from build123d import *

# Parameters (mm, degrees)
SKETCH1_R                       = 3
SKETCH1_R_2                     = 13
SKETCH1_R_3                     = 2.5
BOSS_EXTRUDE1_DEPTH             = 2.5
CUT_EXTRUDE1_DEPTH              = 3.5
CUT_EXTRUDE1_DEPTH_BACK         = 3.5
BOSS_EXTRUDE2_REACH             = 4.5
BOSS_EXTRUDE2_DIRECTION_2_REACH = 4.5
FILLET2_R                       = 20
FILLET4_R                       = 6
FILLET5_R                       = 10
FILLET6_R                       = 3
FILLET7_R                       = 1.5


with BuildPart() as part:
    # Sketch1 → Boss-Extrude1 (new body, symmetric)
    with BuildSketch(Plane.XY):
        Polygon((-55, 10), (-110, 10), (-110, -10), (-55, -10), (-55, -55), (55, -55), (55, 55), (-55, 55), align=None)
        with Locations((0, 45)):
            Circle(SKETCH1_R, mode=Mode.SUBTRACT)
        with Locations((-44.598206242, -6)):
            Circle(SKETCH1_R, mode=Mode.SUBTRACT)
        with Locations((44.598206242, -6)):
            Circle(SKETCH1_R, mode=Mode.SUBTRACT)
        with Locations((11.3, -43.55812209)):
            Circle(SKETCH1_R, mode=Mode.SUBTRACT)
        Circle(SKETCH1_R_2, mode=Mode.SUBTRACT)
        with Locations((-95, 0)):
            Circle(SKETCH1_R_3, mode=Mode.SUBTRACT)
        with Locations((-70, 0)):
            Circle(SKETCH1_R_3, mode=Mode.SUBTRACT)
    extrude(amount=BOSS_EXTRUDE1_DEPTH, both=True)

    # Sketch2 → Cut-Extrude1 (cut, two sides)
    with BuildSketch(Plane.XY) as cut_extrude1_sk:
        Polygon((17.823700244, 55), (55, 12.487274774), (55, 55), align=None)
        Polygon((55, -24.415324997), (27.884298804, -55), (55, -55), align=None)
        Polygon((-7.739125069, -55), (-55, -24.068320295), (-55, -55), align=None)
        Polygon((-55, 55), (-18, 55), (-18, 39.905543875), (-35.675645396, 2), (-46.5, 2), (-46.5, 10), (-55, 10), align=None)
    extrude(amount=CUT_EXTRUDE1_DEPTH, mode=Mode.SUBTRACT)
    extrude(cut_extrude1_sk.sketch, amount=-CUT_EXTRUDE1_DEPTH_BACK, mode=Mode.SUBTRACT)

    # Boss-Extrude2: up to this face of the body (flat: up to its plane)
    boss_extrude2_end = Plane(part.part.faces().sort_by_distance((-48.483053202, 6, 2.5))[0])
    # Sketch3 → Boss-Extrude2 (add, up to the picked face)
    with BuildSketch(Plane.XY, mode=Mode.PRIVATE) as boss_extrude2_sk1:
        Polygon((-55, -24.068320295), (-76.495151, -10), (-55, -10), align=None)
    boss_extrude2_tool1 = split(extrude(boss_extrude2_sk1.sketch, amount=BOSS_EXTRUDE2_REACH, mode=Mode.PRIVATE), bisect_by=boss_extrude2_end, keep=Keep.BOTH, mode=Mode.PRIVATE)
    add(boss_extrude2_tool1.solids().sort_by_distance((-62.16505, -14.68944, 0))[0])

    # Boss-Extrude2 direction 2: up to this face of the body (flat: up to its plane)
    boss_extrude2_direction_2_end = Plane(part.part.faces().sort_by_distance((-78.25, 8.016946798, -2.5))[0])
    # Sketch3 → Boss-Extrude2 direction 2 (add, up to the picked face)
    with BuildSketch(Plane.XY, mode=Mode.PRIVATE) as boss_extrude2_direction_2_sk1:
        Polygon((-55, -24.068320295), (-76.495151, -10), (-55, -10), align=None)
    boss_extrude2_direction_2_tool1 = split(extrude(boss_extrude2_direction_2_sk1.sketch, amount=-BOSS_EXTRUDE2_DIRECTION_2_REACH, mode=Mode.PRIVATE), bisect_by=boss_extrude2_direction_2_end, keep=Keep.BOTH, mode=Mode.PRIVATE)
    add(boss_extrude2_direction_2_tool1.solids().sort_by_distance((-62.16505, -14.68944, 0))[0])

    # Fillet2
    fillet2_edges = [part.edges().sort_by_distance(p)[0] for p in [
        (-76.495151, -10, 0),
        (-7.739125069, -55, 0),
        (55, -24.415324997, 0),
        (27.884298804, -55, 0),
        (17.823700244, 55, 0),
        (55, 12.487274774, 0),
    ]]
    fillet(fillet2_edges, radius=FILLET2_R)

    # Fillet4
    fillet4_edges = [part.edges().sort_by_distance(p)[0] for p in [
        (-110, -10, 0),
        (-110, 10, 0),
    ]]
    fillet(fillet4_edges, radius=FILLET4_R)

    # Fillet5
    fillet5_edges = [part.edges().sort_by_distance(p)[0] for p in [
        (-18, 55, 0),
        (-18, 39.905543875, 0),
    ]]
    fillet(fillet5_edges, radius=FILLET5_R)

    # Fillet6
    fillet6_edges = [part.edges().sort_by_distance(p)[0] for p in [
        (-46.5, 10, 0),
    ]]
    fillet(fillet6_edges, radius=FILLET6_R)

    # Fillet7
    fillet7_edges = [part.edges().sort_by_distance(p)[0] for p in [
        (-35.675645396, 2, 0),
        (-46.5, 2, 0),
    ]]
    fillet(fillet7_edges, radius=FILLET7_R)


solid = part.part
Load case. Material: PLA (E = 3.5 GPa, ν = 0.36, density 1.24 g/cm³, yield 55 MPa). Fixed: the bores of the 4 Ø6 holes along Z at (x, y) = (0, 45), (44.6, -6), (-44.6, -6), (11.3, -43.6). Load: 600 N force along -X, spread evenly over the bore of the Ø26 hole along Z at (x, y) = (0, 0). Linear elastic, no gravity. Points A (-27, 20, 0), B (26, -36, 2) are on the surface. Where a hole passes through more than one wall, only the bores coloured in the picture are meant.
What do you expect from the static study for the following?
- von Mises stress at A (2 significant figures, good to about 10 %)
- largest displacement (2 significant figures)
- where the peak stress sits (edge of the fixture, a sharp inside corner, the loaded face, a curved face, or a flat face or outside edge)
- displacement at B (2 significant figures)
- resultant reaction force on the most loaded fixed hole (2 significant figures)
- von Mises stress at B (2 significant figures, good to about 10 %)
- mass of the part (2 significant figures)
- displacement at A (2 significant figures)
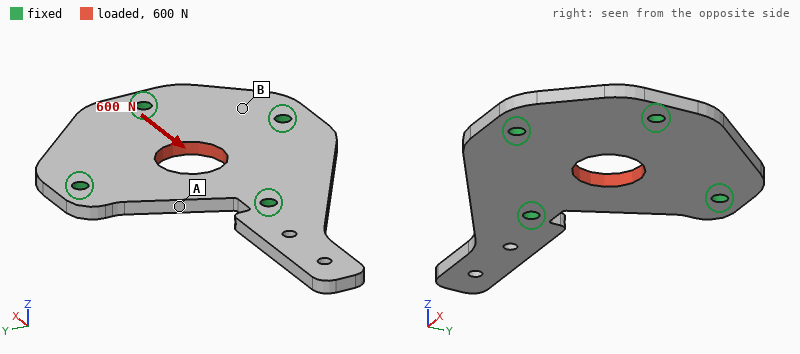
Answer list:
1.7 MPa
26 µm
a curved face
4.5 µm
200 N
0.42 MPa
56 g
20 µm
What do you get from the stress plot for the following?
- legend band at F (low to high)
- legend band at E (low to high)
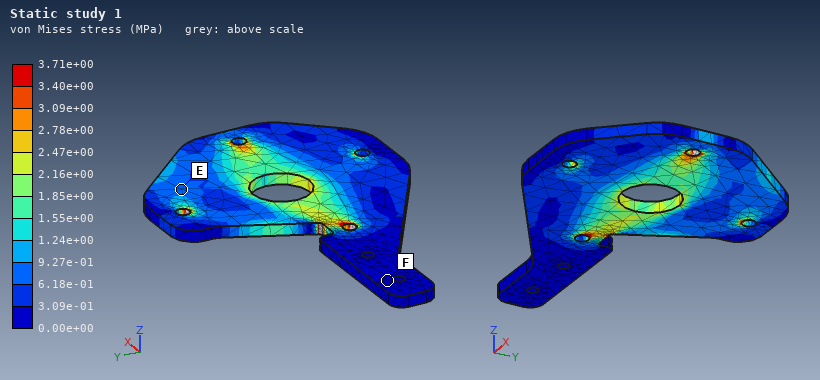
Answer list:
0.00e+00 to 3.09e-01 MPa
6.18e-01 to 9.27e-01 MPa
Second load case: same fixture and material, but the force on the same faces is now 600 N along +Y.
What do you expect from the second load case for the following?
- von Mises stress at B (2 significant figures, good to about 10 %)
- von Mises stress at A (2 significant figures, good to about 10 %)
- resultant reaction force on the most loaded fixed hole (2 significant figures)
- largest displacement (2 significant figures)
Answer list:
0.43 MPa
0.64 MPa
220 N
24 µm
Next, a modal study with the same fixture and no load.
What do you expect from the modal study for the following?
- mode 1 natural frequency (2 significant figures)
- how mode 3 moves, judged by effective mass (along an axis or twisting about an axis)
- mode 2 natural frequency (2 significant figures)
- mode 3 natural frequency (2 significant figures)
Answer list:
380 Hz
along Z
1500 Hz
1600 Hz
